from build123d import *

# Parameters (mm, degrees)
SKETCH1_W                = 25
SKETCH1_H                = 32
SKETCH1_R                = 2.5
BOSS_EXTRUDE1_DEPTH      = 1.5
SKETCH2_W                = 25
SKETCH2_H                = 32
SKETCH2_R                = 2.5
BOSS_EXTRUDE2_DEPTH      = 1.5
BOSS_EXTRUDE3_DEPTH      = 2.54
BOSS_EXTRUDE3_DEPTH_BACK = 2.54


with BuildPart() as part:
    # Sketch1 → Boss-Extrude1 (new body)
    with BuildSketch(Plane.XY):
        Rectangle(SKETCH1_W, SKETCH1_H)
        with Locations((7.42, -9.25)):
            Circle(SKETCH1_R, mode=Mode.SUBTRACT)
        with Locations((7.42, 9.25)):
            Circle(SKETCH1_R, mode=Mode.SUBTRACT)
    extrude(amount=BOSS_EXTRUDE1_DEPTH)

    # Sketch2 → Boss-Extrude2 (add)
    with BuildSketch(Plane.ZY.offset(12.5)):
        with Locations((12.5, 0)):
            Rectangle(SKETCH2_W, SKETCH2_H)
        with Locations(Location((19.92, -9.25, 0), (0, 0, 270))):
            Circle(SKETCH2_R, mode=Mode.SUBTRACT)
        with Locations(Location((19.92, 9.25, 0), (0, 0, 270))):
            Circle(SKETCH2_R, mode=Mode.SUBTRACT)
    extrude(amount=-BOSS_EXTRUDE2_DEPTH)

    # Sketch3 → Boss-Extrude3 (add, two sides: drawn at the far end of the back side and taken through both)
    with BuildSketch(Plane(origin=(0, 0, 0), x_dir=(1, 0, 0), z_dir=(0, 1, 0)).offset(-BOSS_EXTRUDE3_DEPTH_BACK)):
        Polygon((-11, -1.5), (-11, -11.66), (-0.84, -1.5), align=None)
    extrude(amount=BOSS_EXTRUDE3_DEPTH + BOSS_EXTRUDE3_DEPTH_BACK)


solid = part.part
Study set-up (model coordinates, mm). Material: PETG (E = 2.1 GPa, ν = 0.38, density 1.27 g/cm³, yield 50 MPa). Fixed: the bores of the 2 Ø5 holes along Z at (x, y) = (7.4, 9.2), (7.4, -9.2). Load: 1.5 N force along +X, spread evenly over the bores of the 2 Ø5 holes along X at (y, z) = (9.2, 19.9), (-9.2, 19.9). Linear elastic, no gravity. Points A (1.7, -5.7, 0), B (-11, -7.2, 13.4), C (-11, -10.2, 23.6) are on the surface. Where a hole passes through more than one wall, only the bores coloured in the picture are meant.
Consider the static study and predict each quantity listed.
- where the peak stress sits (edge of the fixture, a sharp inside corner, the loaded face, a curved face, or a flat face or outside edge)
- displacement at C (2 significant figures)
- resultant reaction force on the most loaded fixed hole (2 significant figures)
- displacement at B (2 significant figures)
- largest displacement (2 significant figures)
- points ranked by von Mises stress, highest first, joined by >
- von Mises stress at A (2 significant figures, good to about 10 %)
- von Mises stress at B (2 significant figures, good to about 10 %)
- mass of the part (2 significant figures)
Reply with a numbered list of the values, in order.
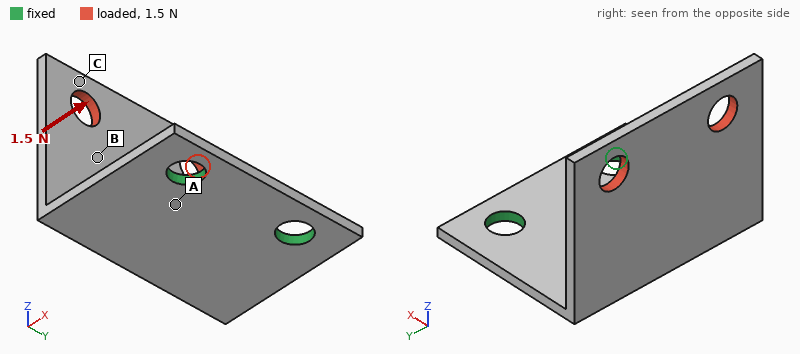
1. a flat face or outside edge
2. 0.40 mm
3. 0.88 N
4. 0.24 mm
5. 0.44 mm
6. A > B > C
7. 2.2 MPa
8. 0.63 MPa
9. 3.1 g
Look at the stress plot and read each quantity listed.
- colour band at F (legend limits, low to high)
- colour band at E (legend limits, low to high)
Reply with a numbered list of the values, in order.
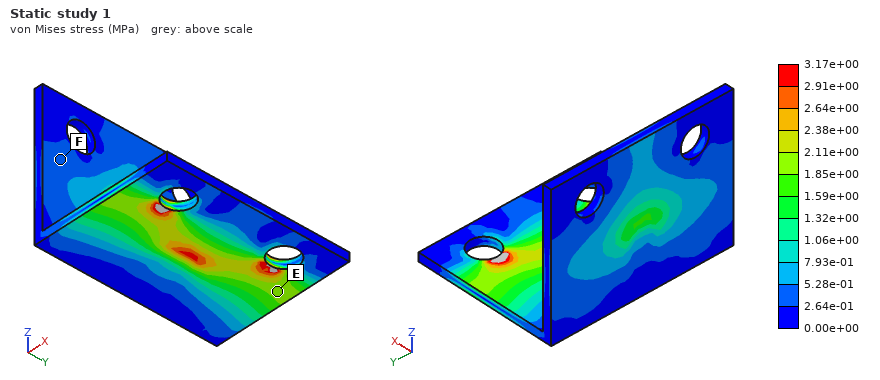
1. 2.64e-01 to 5.28e-01 MPa
2. 1.85e+00 to 2.11e+00 MPa
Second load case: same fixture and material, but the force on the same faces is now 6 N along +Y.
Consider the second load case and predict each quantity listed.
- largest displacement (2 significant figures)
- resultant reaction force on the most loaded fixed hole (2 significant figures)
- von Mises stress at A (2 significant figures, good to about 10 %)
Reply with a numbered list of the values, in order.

1. 0.56 mm
2. 8.7 N
3. 2.4 MPa
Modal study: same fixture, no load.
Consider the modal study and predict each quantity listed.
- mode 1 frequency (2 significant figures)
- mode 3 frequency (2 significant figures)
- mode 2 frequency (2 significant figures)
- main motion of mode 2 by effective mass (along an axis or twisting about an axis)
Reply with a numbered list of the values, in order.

1. 300 Hz
2. 1200 Hz
3. 600 Hz
4. along Y
